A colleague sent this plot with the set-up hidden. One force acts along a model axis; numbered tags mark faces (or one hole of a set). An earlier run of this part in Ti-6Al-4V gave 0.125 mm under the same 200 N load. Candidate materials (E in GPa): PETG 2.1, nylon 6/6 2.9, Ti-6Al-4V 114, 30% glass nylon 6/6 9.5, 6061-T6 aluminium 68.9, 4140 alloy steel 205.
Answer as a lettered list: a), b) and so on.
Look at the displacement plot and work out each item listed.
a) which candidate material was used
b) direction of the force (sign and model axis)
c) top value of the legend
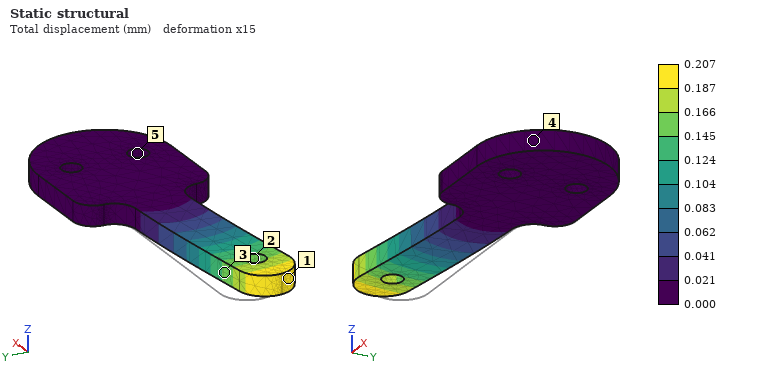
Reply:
a) 6061-T6 aluminium
b) -Y
c) 0.207 mm
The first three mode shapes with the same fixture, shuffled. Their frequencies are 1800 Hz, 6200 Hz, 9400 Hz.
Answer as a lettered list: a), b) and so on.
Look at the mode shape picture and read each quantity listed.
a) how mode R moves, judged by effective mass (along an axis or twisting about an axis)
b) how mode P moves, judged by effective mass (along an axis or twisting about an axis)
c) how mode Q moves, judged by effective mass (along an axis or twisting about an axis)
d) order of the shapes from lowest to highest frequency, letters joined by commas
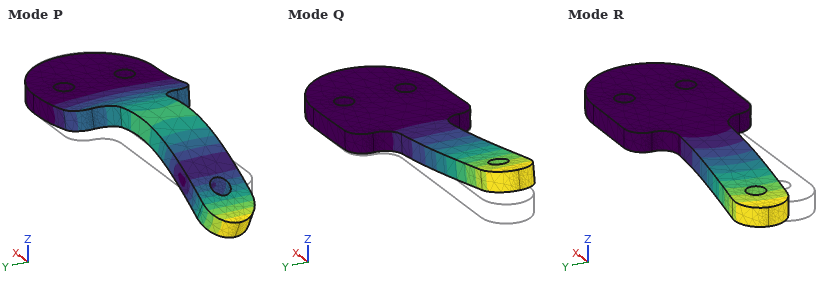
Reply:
a) along Y
b) along Z
c) along Z
d) Q, R, P
